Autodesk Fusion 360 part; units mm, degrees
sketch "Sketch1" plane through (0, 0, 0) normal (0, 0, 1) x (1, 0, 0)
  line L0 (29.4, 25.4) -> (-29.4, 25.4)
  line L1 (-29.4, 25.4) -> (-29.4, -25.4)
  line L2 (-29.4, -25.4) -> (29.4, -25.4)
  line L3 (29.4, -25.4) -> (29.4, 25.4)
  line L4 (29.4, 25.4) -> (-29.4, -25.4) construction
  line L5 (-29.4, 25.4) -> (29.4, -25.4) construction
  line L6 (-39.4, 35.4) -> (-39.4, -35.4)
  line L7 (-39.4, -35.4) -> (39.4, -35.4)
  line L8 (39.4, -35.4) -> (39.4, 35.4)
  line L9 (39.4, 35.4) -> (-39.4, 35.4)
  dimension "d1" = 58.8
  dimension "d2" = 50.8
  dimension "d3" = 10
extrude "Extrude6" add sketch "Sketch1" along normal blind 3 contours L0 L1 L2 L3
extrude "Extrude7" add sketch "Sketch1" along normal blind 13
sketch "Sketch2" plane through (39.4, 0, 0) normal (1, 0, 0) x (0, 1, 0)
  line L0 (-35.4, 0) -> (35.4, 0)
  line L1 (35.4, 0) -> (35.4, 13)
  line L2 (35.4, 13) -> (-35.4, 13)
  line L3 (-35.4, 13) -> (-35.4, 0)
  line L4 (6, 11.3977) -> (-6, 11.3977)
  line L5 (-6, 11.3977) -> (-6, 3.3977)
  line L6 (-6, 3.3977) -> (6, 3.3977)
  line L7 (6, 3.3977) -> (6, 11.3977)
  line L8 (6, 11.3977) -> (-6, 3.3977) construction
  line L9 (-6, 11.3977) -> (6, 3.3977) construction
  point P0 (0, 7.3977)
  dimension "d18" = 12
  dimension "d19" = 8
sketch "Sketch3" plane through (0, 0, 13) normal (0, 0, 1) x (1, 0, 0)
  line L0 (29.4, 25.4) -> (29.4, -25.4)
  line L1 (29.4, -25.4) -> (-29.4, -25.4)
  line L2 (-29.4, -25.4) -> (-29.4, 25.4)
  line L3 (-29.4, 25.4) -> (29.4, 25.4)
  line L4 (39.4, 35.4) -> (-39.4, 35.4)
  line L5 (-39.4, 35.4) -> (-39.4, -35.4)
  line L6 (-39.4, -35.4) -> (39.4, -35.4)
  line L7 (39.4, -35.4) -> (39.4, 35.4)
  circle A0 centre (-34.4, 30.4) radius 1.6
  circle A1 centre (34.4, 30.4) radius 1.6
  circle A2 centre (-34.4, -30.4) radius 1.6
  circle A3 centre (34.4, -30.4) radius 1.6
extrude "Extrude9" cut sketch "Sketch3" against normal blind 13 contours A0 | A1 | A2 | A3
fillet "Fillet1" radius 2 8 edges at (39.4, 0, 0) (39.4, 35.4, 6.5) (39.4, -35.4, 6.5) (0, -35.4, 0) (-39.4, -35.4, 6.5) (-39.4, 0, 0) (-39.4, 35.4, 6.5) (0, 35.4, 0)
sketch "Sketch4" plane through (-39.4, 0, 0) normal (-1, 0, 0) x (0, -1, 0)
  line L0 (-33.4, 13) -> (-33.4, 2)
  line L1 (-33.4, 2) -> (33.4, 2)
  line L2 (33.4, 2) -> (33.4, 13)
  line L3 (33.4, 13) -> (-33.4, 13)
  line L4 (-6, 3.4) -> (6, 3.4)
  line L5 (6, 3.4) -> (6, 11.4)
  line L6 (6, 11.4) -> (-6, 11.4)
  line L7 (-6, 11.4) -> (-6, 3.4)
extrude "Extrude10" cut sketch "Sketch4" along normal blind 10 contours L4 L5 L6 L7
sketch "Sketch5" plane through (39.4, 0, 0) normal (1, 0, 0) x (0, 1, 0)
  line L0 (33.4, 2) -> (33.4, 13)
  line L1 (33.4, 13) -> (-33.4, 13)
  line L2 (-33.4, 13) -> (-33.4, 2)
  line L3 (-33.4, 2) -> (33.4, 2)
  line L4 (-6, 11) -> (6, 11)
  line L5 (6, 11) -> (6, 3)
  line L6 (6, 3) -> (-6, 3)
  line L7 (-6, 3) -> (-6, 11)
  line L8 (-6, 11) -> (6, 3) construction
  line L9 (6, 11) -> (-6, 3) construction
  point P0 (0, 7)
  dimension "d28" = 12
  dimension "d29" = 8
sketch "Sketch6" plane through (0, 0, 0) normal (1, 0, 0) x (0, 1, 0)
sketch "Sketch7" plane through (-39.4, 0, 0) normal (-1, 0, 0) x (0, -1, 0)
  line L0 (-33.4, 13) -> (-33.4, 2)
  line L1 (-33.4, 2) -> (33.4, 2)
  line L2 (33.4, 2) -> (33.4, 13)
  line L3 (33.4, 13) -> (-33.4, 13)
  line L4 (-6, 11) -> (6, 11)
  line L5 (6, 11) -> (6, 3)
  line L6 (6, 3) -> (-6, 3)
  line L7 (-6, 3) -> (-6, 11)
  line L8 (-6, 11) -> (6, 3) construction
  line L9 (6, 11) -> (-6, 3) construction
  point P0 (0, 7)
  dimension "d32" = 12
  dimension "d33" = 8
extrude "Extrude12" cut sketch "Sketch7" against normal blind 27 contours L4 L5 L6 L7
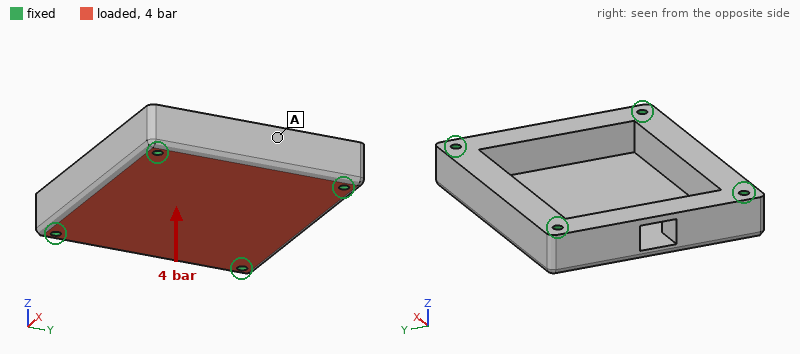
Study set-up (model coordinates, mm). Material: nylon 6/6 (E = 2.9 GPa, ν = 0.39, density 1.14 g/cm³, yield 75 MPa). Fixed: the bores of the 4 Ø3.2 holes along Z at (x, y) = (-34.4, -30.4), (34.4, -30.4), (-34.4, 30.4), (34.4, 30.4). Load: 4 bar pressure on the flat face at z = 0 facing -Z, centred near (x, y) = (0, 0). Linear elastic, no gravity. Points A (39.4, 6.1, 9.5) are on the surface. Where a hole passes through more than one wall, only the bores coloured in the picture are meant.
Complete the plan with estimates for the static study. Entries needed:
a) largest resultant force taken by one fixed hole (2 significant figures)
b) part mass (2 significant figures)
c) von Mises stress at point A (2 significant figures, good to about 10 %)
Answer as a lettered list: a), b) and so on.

a) 570 N
b) 47 g
c) 4.8 MPa
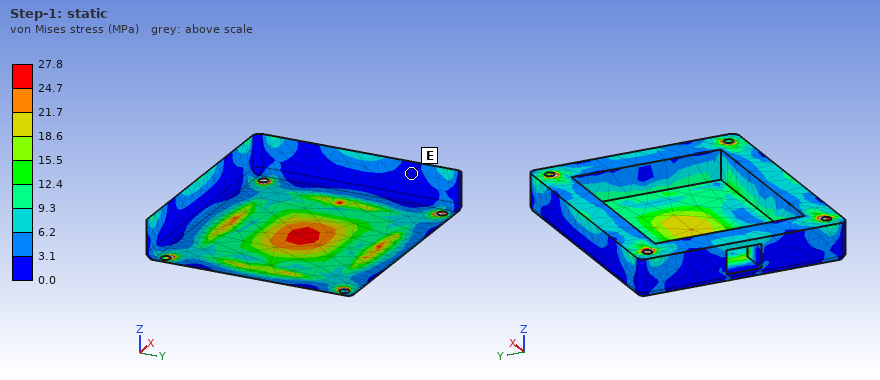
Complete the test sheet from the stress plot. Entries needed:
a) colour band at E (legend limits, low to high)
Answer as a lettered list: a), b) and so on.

a) 0.0 to 3.1 MPa
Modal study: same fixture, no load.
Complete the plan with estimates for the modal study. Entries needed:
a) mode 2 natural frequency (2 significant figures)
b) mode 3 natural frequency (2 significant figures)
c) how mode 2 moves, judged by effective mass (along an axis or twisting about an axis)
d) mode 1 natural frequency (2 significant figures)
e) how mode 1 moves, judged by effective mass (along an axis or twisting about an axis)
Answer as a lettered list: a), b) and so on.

a) 3300 Hz
b) 3700 Hz
c) twisting about X
d) 2100 Hz
e) along Z
